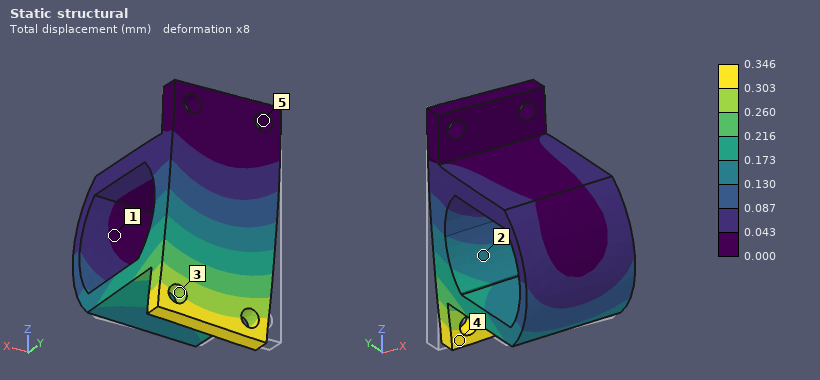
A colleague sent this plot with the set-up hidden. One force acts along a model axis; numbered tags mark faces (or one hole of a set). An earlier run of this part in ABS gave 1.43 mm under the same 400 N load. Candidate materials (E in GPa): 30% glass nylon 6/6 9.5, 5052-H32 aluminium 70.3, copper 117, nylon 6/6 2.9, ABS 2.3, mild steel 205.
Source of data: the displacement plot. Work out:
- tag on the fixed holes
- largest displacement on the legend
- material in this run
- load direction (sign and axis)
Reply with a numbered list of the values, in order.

1. 5
2. 0.346 mm
3. 30% glass nylon 6/6
4. +X
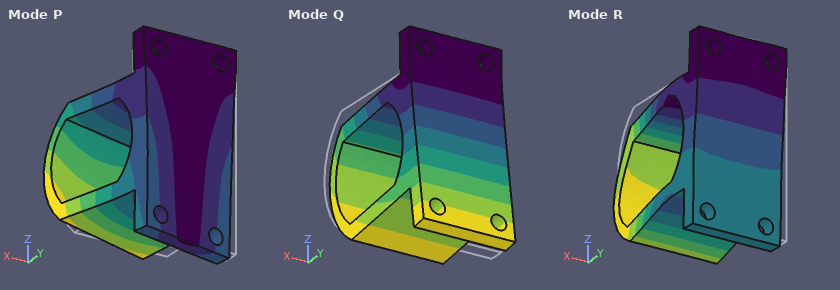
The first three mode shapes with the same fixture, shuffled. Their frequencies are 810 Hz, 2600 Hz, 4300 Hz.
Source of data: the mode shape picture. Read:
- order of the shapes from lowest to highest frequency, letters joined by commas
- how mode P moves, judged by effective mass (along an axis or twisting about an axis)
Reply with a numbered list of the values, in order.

1. Q, P, R
2. along X
